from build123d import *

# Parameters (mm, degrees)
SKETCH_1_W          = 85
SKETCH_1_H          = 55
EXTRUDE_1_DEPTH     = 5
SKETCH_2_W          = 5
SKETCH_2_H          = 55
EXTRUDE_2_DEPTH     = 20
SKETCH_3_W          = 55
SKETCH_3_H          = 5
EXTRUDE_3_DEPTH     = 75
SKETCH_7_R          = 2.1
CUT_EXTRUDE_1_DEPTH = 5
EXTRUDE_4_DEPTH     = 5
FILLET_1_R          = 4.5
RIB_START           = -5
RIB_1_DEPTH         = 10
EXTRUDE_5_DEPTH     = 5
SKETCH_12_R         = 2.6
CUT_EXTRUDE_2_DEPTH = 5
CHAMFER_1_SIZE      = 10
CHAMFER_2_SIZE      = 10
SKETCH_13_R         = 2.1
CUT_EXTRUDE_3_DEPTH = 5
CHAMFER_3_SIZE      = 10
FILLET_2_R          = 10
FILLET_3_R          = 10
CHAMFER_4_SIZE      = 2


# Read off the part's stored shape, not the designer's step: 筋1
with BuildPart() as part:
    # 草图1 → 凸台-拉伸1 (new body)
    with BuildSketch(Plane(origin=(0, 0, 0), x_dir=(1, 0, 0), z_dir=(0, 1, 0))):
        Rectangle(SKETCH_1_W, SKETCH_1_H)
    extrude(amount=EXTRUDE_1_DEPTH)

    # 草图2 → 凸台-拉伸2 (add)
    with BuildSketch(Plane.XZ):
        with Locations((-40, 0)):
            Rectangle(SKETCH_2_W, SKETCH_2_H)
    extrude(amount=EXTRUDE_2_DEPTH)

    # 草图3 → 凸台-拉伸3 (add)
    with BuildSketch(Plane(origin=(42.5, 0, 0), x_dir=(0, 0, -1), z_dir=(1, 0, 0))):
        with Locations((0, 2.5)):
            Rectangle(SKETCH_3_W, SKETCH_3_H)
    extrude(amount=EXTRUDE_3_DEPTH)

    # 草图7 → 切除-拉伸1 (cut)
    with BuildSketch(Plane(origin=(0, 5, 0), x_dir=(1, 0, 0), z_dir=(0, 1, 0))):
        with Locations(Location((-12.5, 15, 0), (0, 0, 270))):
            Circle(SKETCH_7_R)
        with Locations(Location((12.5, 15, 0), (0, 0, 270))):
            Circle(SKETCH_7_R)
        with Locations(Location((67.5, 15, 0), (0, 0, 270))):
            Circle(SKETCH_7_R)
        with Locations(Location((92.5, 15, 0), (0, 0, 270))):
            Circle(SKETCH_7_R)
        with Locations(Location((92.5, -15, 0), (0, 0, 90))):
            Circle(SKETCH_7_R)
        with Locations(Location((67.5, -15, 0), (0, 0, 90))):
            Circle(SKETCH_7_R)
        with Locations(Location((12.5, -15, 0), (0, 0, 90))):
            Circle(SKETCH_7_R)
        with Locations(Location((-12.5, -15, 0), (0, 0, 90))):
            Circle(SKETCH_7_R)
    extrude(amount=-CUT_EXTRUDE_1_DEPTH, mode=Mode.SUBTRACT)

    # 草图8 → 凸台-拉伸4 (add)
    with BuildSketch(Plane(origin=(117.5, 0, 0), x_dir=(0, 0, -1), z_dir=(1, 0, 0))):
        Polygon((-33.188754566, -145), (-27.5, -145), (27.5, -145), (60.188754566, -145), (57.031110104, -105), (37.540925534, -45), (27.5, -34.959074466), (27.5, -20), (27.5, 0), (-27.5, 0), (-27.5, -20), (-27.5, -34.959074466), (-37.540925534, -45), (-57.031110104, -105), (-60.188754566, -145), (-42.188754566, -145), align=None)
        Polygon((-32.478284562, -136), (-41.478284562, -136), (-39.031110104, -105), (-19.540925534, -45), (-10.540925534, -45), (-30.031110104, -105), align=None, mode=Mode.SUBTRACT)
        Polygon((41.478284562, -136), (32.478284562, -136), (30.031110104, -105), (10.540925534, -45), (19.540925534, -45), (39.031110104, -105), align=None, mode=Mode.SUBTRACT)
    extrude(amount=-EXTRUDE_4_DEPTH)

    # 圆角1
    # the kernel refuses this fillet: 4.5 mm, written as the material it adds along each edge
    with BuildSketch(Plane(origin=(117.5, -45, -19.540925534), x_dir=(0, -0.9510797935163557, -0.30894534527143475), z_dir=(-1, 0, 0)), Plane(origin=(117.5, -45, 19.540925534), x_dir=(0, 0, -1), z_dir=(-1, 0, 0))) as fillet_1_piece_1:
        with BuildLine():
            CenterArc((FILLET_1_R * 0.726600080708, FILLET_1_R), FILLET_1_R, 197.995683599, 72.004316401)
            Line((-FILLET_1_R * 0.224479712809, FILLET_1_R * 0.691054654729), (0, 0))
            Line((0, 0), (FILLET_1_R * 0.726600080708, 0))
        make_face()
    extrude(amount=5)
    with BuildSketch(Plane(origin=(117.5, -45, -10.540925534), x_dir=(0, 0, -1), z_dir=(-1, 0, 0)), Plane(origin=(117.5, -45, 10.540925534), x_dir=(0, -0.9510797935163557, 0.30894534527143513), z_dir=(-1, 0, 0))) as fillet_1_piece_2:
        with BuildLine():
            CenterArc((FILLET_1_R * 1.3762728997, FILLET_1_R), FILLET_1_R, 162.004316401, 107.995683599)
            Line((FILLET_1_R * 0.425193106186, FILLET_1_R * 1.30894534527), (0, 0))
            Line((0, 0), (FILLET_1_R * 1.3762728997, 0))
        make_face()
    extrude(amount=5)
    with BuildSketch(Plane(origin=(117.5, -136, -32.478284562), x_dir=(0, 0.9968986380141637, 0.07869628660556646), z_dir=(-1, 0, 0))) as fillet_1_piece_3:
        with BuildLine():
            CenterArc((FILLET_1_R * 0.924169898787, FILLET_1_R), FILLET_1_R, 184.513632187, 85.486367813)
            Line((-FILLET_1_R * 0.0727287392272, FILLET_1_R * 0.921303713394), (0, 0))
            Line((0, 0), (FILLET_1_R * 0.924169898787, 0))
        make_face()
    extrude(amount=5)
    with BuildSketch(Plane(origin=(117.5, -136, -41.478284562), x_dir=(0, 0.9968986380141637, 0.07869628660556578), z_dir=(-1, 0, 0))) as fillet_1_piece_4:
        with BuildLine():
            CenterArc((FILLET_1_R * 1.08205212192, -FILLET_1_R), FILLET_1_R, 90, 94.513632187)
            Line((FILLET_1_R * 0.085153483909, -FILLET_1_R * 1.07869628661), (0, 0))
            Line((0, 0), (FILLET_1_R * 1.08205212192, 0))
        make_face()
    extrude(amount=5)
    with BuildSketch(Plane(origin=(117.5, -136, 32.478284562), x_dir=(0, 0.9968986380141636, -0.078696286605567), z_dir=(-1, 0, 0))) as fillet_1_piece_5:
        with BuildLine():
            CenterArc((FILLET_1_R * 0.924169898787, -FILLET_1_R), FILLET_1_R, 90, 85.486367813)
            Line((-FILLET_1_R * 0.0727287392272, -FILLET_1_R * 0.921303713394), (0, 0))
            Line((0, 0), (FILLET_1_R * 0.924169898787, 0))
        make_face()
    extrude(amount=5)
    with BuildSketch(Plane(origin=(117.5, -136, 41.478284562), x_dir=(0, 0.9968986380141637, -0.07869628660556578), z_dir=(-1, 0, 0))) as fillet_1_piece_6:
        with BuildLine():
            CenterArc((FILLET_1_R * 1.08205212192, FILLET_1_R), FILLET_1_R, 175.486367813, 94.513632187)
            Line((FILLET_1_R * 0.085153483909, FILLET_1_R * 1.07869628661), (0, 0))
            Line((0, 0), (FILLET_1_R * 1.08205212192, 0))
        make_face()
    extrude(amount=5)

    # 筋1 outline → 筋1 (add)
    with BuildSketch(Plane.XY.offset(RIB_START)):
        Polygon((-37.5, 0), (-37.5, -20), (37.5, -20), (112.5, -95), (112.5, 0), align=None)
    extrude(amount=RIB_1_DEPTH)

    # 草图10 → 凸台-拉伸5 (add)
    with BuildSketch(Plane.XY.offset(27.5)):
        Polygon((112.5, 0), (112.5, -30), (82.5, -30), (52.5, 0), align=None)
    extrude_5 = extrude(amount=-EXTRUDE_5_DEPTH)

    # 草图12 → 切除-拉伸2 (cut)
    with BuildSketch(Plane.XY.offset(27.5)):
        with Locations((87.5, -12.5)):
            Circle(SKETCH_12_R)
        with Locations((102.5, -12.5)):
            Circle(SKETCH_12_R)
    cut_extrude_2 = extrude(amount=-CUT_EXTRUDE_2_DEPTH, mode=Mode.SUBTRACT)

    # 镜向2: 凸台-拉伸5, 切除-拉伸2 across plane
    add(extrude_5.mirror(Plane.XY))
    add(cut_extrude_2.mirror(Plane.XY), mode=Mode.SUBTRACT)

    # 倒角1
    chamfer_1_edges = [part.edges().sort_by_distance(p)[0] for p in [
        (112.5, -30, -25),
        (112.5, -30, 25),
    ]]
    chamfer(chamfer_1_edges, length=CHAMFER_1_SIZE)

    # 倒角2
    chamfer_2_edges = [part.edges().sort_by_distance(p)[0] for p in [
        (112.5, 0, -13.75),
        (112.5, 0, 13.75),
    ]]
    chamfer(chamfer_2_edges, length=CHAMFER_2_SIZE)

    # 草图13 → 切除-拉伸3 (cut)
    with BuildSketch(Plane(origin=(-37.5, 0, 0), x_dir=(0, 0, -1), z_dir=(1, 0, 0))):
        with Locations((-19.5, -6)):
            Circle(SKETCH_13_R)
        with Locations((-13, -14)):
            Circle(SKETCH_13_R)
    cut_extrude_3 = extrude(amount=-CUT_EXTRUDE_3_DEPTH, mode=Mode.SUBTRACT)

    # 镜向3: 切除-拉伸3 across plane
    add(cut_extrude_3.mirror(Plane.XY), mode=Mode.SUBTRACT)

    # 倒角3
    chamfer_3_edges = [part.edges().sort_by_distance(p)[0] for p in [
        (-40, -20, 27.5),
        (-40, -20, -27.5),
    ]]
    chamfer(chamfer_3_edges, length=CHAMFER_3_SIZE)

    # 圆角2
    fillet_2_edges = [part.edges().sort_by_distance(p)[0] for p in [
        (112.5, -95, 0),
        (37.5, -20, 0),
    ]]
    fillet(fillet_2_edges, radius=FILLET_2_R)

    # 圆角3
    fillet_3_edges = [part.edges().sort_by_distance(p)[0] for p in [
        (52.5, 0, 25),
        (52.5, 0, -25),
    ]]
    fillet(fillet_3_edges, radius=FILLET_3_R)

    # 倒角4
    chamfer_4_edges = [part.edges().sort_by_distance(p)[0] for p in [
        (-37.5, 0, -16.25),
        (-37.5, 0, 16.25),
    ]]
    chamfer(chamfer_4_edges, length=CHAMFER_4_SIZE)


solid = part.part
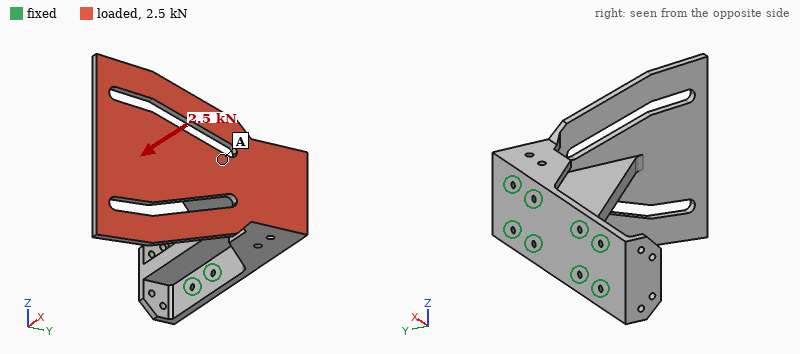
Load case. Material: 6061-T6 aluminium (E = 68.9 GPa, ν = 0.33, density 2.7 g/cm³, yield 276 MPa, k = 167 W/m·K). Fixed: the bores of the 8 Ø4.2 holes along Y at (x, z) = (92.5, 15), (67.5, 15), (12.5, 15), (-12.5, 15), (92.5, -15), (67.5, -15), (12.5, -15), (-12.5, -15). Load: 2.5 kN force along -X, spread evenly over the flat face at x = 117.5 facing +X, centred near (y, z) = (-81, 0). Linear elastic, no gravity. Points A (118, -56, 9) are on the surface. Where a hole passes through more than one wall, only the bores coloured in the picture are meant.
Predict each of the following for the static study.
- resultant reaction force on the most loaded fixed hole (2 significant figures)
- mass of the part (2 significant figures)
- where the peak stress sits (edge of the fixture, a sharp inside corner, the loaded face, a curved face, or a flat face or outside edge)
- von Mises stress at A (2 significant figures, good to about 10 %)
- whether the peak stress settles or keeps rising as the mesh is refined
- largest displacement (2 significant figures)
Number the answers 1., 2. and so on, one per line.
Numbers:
1. 1.8 kN
2. 480 g
3. a sharp inside corner
4. 24 MPa
5. keeps rising
6. 1.3 mm
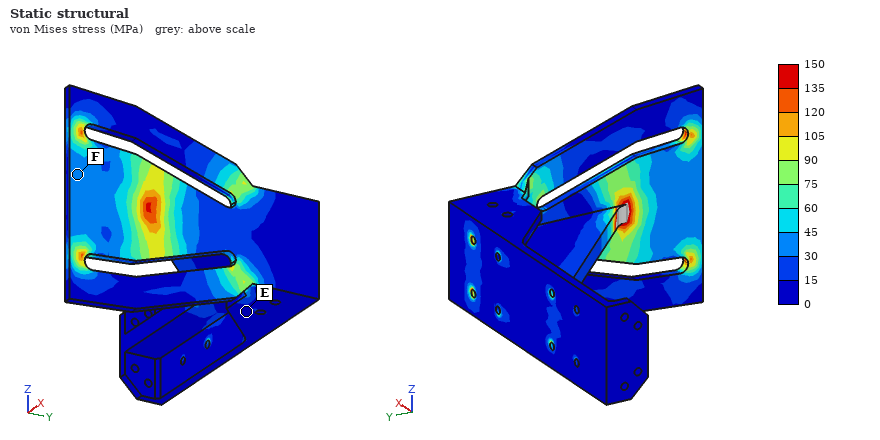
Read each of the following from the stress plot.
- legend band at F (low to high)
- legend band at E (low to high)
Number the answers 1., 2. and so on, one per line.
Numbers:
1. 30 to 45 MPa
2. 0 to 15 MPa
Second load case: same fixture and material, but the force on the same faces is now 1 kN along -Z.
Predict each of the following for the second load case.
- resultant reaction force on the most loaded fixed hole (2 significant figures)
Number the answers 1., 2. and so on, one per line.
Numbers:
1. 2.2 kN
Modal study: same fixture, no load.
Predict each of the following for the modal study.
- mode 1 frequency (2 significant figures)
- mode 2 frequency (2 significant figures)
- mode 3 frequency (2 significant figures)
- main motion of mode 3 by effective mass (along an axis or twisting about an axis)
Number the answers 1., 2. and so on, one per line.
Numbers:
1. 710 Hz
2. 720 Hz
3. 760 Hz
4. along Z
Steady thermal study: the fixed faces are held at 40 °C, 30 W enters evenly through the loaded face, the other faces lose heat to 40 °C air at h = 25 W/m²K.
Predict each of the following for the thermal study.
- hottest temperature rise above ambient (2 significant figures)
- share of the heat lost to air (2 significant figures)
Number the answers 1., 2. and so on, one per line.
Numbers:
1. 21 K
2. 26 %
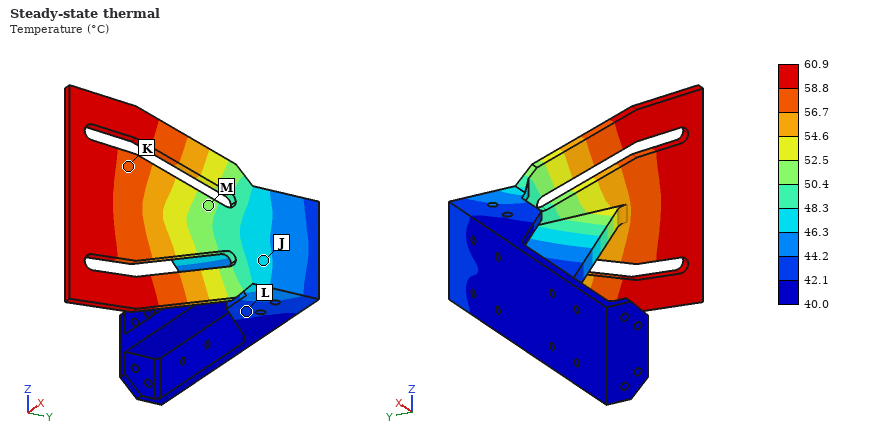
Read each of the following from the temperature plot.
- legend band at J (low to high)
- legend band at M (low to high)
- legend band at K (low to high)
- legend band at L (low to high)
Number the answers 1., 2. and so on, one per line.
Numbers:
1. 46.3 to 48.3 °C
2. 50.4 to 52.5 °C
3. 56.7 to 58.8 °C
4. 42.1 to 44.2 °C
